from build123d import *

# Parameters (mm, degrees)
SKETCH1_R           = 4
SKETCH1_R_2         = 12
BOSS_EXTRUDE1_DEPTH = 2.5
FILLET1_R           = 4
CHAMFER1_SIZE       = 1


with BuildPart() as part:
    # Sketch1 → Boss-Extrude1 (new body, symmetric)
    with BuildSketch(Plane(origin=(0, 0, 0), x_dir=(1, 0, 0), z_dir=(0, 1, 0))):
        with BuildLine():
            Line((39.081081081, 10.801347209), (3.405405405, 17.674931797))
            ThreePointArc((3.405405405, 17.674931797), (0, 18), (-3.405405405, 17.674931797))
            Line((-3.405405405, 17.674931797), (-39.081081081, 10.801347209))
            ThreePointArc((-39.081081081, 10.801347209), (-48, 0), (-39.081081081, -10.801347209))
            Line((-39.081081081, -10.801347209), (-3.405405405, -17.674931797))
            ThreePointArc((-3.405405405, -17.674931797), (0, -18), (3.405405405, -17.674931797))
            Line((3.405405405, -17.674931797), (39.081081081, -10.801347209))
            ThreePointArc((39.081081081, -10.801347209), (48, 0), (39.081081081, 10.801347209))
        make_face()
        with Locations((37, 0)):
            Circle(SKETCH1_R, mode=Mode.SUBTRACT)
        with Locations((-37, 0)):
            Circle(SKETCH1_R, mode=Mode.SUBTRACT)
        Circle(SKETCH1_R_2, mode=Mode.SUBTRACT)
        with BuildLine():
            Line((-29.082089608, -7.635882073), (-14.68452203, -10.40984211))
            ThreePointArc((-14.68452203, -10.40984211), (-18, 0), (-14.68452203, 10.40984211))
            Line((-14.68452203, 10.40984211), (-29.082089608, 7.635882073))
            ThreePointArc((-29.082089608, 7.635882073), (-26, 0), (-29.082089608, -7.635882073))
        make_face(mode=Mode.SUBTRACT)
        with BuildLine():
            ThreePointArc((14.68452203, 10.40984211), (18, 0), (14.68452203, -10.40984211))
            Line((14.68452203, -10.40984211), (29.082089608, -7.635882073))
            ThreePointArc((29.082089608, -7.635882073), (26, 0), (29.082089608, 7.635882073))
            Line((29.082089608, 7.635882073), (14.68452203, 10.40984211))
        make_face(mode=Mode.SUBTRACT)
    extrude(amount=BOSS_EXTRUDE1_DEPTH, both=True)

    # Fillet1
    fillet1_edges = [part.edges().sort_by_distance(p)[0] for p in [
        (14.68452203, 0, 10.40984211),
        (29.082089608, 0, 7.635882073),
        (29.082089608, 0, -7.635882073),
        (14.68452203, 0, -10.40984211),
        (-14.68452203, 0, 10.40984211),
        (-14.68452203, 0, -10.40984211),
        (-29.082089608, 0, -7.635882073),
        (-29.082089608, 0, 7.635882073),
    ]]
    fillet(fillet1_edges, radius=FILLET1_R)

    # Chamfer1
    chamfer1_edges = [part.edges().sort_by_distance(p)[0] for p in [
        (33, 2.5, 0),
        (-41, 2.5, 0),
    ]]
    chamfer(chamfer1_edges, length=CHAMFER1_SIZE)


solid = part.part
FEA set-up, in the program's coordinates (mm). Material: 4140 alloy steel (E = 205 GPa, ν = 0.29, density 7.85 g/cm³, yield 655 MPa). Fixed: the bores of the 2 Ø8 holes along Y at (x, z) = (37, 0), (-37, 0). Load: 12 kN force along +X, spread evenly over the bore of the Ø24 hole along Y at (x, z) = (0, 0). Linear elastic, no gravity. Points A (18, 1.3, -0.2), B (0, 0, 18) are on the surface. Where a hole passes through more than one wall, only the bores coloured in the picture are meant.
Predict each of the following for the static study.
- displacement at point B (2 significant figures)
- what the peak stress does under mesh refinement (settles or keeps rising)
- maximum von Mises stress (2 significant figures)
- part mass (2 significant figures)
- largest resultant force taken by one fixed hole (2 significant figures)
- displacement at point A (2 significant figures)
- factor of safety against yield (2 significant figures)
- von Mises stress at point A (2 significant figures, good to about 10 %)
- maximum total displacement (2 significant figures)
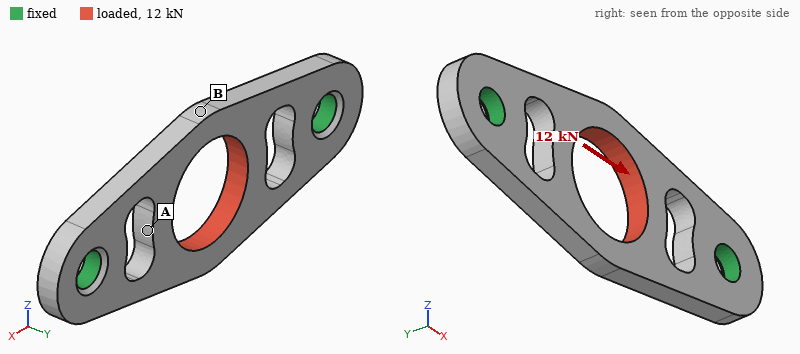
16 µm
settles
320 MPa
67 g
6.0 kN
22 µm
2.1
110 MPa
23 µm
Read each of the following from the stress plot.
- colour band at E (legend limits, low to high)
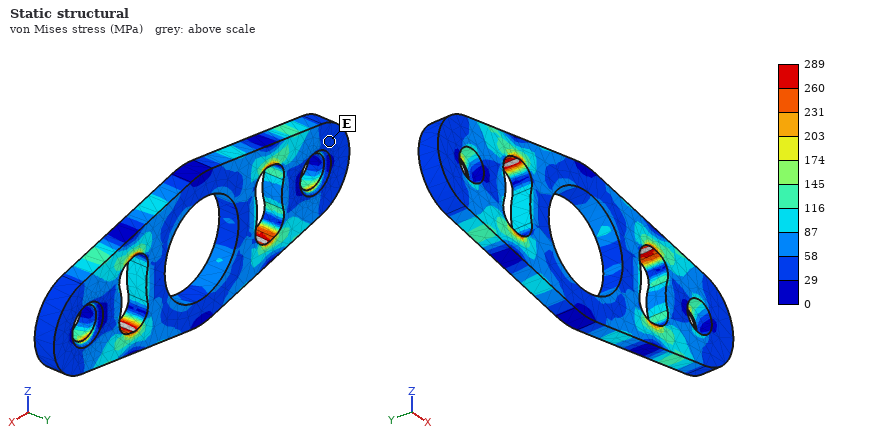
29 to 58 MPa
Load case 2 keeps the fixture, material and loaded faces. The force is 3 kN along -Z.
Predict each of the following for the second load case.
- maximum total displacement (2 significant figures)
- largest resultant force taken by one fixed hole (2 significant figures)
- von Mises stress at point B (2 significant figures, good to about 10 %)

22 µm
1.5 kN
48 MPa
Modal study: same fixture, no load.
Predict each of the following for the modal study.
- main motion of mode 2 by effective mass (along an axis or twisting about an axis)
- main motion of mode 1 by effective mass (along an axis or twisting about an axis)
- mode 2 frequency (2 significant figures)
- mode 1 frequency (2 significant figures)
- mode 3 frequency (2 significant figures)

twisting about X
along Y
5300 Hz
4400 Hz
11 kHz
